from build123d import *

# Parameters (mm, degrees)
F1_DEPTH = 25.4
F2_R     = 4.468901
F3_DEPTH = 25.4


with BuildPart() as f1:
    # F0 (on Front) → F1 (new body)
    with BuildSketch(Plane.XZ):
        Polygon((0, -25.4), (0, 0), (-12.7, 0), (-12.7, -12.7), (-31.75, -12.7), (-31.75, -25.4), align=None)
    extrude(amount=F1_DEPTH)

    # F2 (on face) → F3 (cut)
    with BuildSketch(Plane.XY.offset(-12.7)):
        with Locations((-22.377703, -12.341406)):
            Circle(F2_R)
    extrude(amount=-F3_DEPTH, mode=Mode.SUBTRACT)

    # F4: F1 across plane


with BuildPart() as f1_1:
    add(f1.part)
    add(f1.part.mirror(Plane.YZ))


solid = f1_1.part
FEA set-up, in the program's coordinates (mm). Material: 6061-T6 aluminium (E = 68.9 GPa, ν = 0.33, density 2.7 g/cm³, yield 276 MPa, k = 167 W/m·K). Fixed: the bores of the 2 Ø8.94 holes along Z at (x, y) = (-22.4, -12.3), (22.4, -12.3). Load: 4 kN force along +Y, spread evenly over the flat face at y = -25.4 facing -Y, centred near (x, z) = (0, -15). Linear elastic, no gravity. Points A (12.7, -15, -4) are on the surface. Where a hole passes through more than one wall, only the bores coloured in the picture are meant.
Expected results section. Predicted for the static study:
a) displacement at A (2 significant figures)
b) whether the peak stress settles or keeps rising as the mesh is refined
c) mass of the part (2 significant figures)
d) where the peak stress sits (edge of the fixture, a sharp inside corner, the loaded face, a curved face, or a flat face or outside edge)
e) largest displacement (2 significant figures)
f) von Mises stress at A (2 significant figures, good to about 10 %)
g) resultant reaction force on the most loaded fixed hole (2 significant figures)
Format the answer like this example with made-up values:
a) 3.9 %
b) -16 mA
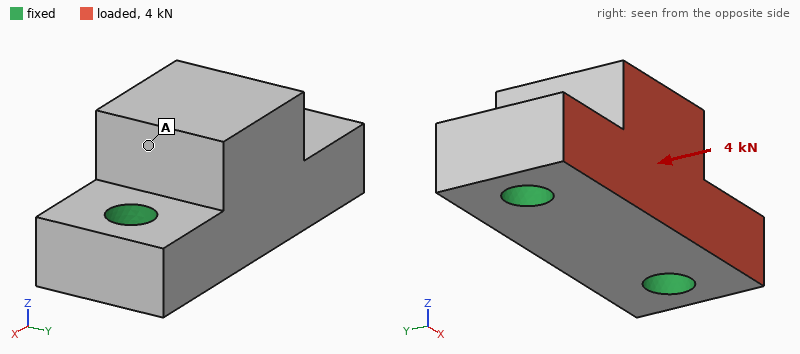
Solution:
a) 6.9 µm
b) keeps rising
c) 73 g
d) edge of the fixture
e) 9.5 µm
f) 3.8 MPa
g) 2.0 kN
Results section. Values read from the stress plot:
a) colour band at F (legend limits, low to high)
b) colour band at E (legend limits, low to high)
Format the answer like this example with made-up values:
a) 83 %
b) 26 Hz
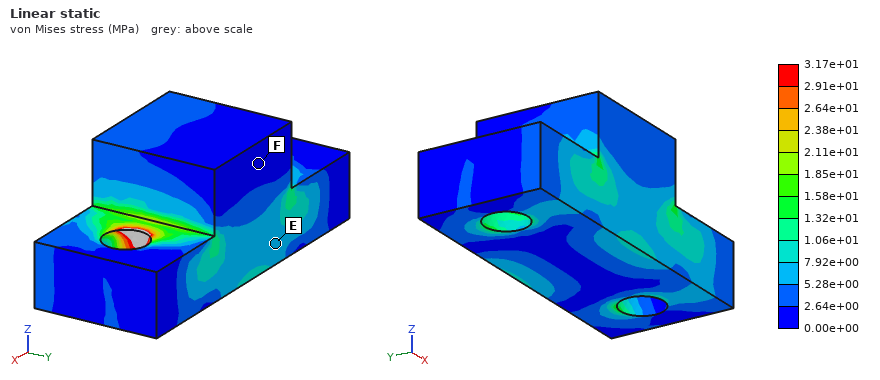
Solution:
a) 0.00e+00 to 2.64e+00 MPa
b) 5.28e+00 to 7.92e+00 MPa
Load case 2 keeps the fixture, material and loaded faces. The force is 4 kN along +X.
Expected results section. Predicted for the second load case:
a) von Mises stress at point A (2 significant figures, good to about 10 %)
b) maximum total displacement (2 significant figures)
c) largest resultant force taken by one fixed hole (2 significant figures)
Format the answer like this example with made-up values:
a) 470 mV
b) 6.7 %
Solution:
a) 4.0 MPa
b) 5.9 µm
c) 2.2 kN
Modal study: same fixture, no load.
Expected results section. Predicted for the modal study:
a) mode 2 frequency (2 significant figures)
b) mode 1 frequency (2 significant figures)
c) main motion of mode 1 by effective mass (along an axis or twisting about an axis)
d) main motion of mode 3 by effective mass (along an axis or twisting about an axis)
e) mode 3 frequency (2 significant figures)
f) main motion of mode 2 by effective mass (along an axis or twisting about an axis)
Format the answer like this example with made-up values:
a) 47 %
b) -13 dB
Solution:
a) 21 kHz
b) 14 kHz
c) along Y
d) along X
e) 27 kHz
f) along Z
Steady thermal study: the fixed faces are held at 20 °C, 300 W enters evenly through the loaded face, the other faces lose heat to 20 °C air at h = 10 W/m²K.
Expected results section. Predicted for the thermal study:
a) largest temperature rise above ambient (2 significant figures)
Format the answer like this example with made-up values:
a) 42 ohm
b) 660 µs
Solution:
a) 44 K
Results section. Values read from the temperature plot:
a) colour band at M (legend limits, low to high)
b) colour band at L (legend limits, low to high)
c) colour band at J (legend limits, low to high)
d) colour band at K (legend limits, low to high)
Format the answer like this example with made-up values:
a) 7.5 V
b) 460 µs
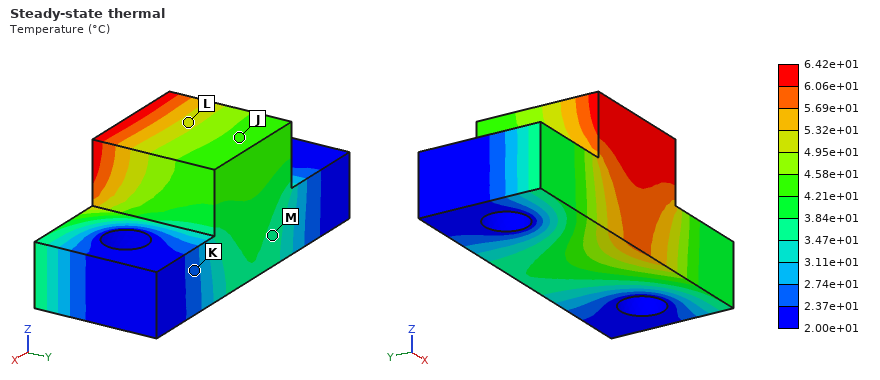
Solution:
a) 3.47e+01 to 3.84e+01 °C
b) 4.95e+01 to 5.32e+01 °C
c) 4.21e+01 to 4.58e+01 °C
d) 2.37e+01 to 2.74e+01 °C
